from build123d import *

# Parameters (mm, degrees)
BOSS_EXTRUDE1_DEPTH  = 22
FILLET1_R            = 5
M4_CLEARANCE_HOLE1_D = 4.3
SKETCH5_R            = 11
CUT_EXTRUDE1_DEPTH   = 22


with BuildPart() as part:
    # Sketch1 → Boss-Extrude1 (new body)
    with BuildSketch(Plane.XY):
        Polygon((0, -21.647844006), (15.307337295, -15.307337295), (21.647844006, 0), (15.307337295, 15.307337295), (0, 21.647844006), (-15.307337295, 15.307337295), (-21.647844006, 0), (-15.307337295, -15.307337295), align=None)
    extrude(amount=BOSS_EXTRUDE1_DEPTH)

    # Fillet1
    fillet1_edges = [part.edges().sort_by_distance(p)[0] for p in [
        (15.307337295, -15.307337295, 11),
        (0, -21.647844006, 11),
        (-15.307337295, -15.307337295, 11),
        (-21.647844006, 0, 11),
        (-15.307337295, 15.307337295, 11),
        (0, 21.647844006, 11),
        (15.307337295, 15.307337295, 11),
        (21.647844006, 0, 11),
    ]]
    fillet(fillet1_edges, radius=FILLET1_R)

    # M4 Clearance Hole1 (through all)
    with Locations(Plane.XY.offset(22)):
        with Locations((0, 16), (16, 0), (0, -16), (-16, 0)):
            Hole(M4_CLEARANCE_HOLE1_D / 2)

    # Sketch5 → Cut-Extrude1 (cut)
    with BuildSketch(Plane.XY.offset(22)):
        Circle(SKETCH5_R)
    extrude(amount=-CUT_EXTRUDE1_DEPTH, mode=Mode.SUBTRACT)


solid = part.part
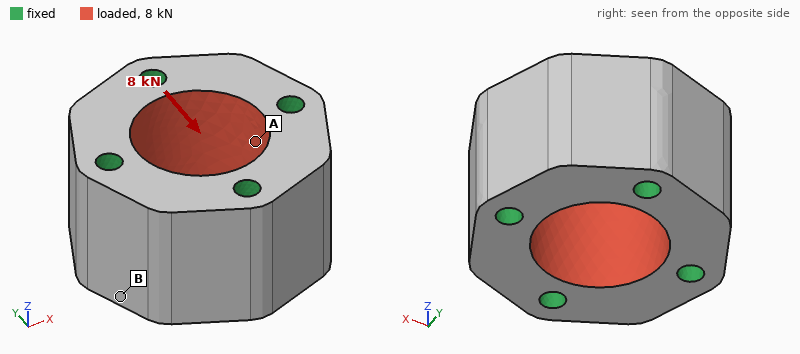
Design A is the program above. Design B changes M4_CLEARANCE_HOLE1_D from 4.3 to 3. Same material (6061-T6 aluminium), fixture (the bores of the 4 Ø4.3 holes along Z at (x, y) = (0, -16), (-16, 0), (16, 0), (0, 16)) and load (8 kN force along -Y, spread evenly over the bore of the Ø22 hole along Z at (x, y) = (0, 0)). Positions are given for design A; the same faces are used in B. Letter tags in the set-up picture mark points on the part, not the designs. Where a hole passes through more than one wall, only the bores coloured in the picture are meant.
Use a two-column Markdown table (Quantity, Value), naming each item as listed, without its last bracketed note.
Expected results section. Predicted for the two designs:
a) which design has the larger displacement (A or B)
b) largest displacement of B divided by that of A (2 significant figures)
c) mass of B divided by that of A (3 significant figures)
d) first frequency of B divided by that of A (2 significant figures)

| Quantity | Value |
|---|---|
| which design has the larger displacement | B |
| largest displacement of B divided by that of A | 1.1 |
| mass of B divided by that of A | 1.03 |
| first frequency of B divided by that of A | 0.90 |
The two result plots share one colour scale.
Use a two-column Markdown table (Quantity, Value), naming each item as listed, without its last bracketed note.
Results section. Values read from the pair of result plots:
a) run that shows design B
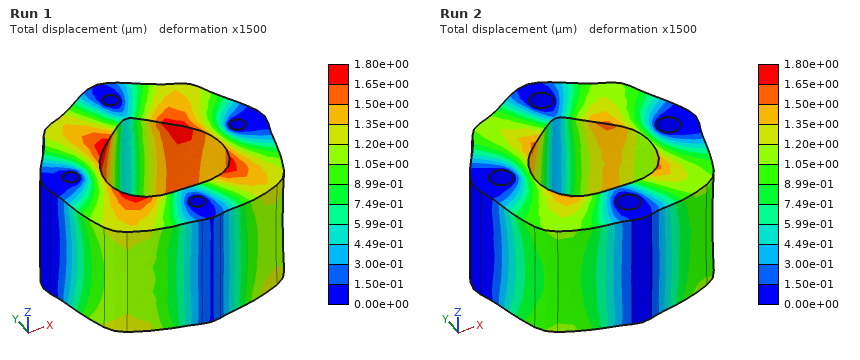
| Quantity | Value |
|---|---|
| run that shows design B | Run 1 |
